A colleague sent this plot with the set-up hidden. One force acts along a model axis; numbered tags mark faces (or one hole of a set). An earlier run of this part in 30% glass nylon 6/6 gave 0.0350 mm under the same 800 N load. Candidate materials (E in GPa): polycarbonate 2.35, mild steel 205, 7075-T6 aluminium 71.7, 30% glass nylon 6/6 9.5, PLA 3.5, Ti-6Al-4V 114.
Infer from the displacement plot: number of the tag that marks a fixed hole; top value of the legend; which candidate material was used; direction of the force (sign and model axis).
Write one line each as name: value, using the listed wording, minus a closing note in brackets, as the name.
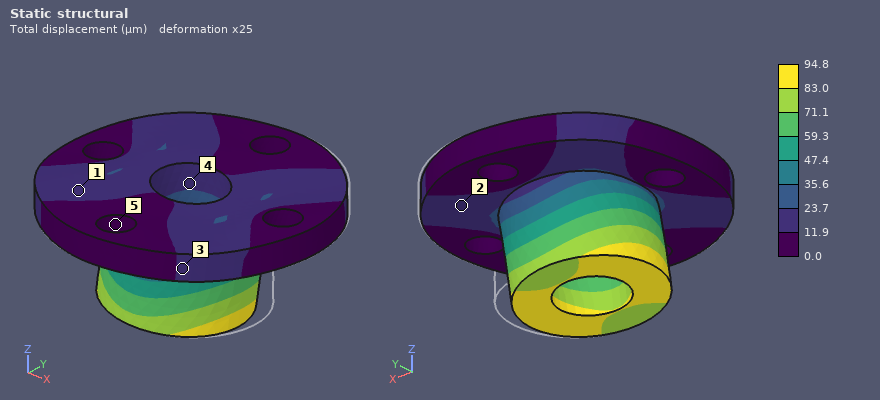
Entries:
number of the tag that marks a fixed hole: 5
top value of the legend: 94.8 µm
which candidate material was used: PLA
direction of the force: -X
